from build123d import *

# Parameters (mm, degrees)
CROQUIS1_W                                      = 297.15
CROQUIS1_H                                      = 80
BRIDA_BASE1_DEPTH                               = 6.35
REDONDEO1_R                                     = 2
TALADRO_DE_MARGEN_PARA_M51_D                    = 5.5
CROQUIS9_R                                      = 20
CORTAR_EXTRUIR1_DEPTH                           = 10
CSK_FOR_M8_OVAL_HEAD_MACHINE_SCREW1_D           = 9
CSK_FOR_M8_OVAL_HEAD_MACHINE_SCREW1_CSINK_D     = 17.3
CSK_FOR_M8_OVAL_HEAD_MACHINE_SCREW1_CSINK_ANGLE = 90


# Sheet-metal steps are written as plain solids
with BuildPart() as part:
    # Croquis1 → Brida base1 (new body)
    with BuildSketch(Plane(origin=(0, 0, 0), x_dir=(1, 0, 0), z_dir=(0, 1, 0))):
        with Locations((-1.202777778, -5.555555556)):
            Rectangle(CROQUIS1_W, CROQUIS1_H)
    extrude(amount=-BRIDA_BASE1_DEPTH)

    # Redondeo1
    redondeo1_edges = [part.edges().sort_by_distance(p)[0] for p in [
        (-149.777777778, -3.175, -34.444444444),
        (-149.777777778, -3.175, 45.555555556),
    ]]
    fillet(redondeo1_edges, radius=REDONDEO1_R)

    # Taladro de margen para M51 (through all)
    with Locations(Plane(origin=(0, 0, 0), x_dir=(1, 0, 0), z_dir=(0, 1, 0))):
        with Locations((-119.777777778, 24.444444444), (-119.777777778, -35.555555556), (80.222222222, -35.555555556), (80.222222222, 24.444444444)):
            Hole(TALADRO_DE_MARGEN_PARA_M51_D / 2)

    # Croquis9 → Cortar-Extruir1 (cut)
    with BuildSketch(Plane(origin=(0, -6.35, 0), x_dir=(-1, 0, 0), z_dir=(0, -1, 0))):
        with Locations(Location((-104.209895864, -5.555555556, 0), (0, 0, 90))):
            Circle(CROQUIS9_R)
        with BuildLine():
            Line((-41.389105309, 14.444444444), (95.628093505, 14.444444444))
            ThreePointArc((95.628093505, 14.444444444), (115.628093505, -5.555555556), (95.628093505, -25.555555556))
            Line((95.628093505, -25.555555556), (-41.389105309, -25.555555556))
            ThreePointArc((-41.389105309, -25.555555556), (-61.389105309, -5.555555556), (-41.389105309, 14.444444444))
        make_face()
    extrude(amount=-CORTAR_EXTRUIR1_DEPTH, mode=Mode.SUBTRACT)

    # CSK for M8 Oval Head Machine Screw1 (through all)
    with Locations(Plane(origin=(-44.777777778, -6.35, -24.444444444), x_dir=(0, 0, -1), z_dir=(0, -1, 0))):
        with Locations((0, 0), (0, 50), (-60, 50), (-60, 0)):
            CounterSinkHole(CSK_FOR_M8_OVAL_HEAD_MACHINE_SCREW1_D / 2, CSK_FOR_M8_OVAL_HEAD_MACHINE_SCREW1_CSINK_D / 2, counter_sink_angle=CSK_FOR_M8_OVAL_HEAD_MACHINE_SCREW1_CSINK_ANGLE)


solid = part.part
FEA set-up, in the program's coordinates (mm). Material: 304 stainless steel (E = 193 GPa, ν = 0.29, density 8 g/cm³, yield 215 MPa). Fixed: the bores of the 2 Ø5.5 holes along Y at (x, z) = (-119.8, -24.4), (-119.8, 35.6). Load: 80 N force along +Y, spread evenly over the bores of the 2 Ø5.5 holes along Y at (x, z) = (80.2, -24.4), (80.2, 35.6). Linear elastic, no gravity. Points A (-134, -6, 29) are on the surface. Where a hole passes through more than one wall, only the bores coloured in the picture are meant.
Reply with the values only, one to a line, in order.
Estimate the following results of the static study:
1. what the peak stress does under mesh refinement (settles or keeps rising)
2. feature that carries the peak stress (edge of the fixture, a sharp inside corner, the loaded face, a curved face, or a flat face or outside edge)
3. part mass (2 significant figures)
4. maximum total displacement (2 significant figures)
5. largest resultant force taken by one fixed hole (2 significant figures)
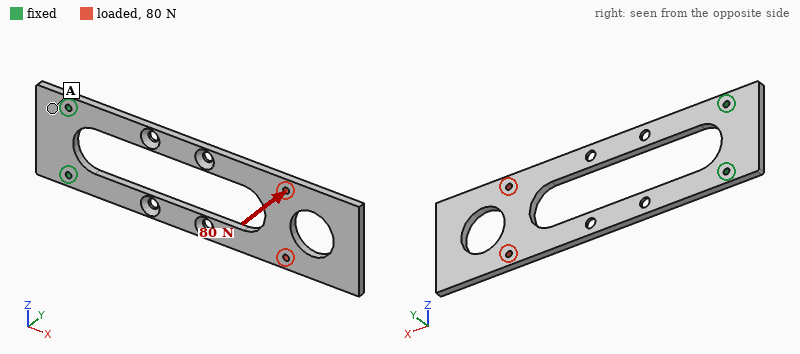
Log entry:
keeps rising
a sharp inside corner
770 g
2.2 mm
40 N
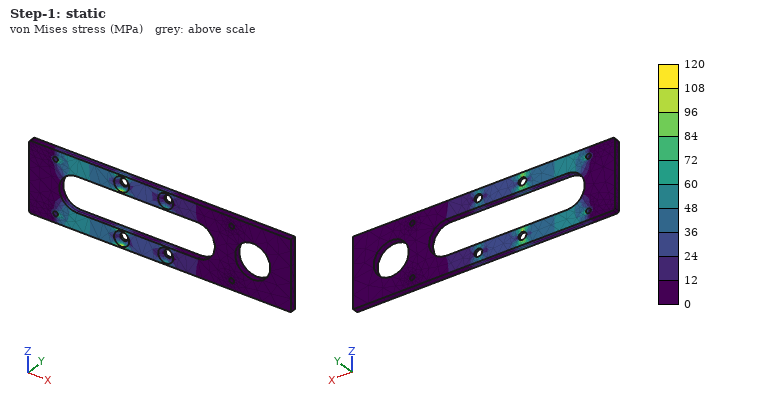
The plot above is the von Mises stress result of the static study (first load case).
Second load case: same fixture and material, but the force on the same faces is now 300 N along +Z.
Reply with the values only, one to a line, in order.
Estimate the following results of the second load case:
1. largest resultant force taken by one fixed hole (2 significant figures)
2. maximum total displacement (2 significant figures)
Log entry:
920 N
0.12 mm
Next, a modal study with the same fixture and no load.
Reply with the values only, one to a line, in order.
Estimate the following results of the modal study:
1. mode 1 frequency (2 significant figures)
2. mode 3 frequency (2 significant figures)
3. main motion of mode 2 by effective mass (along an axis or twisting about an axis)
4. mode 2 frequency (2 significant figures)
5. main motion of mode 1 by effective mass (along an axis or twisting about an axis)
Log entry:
54 Hz
400 Hz
twisting about X
310 Hz
along Y
